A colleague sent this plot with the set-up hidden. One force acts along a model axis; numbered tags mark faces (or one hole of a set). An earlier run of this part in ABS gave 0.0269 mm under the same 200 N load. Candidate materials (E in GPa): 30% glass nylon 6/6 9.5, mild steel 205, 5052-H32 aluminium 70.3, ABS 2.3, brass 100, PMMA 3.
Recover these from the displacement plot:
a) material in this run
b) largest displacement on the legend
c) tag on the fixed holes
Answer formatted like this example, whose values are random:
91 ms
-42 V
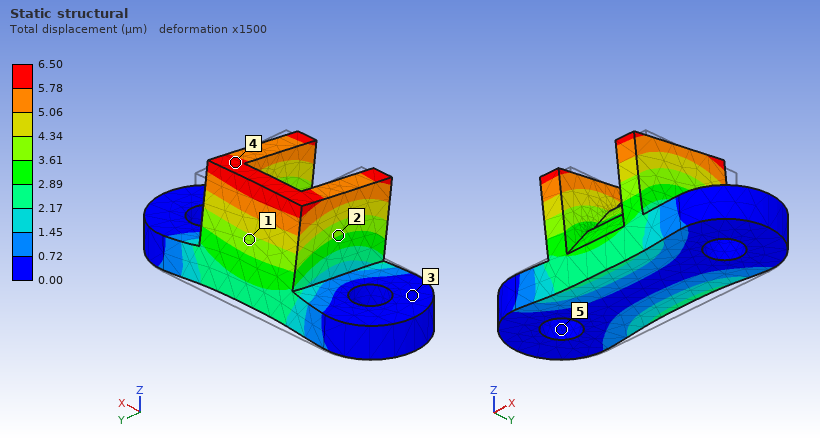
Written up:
30% glass nylon 6/6
6.50 µm
5
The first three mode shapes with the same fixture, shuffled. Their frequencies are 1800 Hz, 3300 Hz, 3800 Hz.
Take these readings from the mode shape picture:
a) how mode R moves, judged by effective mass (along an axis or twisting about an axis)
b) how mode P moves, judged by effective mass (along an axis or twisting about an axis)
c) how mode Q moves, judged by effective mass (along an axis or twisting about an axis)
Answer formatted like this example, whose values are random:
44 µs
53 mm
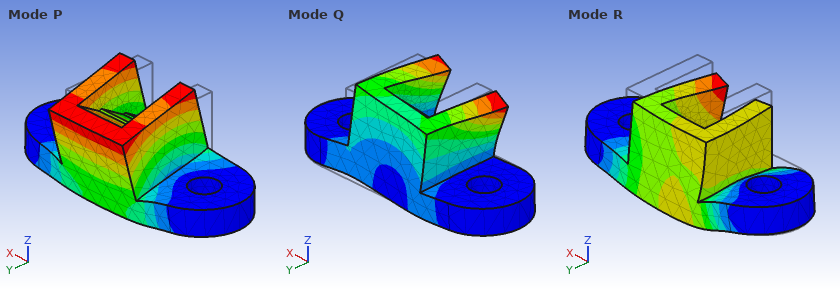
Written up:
along Z
along Y
along X
